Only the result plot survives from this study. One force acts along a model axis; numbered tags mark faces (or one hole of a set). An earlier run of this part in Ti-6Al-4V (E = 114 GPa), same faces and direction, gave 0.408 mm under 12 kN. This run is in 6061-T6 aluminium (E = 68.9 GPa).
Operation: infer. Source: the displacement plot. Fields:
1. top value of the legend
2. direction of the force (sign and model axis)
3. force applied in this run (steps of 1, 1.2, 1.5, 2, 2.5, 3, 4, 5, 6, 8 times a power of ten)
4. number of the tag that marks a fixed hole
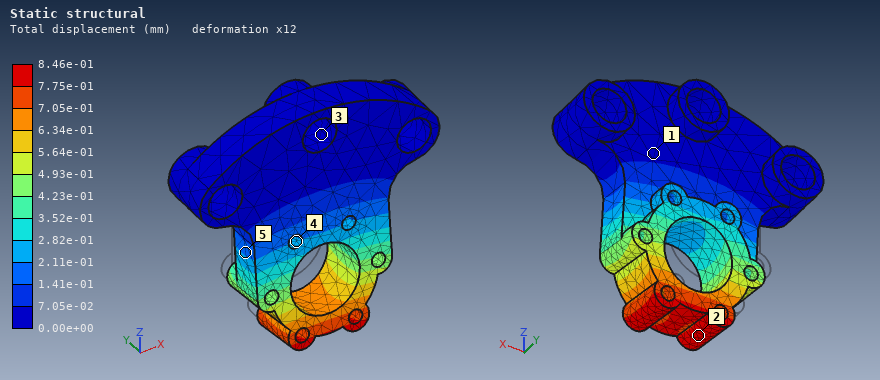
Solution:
8.46e-01 mm
-Y
15 kN
3
